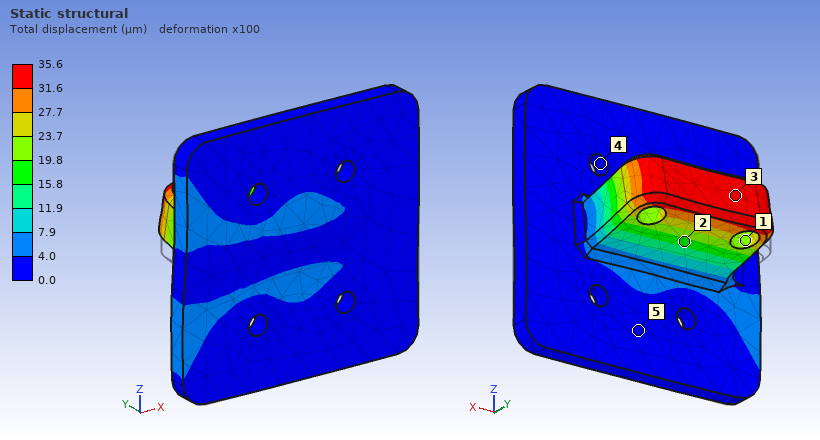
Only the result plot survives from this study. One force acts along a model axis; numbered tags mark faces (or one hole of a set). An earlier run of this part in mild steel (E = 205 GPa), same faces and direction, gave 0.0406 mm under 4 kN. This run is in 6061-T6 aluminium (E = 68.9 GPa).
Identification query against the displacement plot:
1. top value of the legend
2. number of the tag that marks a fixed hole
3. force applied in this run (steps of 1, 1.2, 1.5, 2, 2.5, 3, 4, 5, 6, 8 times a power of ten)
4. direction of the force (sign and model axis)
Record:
35.6 µm
4
1.2 kN
+Z
